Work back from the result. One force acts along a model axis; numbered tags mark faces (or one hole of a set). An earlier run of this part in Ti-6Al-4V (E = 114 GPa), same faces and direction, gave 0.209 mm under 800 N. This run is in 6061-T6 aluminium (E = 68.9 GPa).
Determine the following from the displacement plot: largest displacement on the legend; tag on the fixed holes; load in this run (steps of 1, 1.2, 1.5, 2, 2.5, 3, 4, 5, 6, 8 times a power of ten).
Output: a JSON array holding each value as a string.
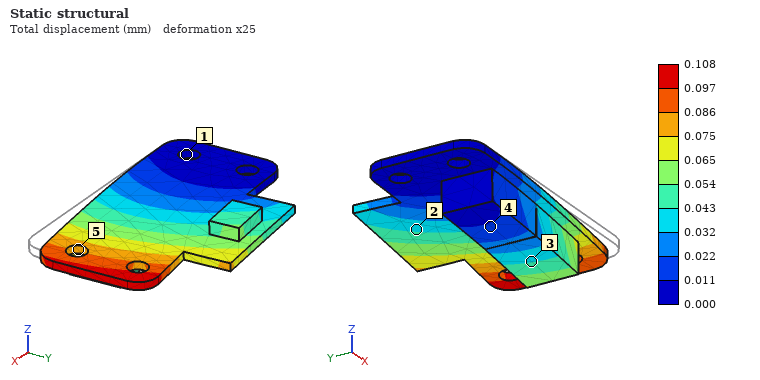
["0.108 mm", "1", "250 N"]
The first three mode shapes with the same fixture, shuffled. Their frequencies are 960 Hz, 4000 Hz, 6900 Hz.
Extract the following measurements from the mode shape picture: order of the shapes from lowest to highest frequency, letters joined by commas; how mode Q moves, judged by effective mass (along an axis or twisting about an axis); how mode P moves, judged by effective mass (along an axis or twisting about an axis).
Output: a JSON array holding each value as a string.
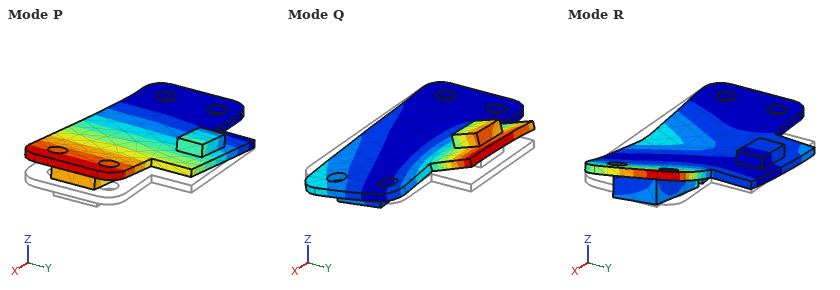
["P, Q, R", "twisting about X", "along Z"]
